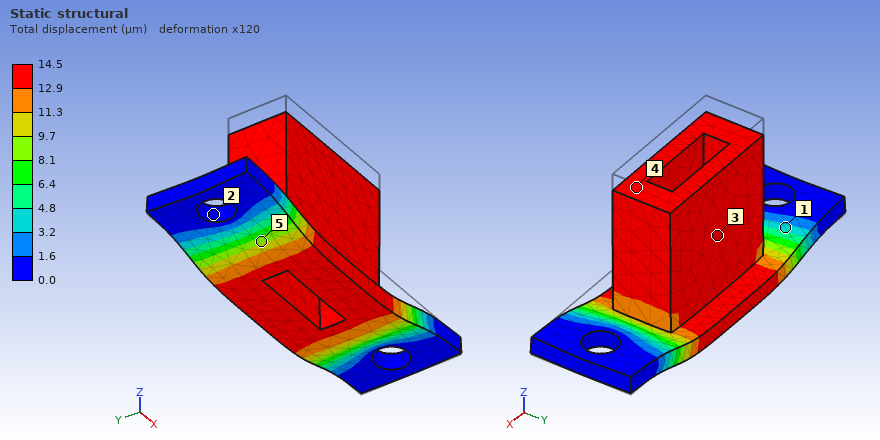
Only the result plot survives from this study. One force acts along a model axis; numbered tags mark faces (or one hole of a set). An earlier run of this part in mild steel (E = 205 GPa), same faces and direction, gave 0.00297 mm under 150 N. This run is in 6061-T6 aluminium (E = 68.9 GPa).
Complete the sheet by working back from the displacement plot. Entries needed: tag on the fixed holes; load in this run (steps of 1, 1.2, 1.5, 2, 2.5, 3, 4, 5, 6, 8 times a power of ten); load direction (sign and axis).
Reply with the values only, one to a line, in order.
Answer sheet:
2
250 N
-Z
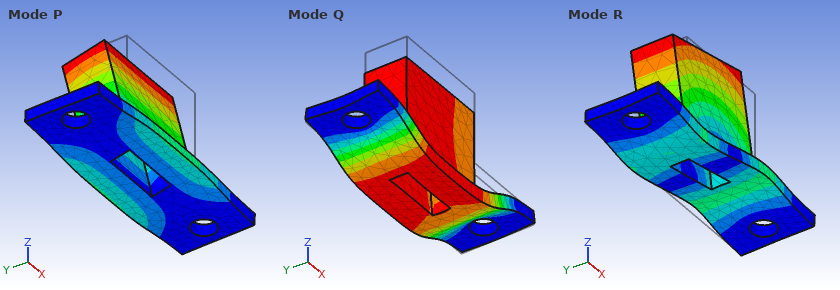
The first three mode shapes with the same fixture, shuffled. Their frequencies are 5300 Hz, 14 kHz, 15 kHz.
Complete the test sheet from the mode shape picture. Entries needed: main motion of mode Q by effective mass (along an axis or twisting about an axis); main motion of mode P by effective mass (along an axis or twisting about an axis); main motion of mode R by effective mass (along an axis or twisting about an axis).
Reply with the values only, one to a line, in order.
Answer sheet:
along Z
along Y
along X
